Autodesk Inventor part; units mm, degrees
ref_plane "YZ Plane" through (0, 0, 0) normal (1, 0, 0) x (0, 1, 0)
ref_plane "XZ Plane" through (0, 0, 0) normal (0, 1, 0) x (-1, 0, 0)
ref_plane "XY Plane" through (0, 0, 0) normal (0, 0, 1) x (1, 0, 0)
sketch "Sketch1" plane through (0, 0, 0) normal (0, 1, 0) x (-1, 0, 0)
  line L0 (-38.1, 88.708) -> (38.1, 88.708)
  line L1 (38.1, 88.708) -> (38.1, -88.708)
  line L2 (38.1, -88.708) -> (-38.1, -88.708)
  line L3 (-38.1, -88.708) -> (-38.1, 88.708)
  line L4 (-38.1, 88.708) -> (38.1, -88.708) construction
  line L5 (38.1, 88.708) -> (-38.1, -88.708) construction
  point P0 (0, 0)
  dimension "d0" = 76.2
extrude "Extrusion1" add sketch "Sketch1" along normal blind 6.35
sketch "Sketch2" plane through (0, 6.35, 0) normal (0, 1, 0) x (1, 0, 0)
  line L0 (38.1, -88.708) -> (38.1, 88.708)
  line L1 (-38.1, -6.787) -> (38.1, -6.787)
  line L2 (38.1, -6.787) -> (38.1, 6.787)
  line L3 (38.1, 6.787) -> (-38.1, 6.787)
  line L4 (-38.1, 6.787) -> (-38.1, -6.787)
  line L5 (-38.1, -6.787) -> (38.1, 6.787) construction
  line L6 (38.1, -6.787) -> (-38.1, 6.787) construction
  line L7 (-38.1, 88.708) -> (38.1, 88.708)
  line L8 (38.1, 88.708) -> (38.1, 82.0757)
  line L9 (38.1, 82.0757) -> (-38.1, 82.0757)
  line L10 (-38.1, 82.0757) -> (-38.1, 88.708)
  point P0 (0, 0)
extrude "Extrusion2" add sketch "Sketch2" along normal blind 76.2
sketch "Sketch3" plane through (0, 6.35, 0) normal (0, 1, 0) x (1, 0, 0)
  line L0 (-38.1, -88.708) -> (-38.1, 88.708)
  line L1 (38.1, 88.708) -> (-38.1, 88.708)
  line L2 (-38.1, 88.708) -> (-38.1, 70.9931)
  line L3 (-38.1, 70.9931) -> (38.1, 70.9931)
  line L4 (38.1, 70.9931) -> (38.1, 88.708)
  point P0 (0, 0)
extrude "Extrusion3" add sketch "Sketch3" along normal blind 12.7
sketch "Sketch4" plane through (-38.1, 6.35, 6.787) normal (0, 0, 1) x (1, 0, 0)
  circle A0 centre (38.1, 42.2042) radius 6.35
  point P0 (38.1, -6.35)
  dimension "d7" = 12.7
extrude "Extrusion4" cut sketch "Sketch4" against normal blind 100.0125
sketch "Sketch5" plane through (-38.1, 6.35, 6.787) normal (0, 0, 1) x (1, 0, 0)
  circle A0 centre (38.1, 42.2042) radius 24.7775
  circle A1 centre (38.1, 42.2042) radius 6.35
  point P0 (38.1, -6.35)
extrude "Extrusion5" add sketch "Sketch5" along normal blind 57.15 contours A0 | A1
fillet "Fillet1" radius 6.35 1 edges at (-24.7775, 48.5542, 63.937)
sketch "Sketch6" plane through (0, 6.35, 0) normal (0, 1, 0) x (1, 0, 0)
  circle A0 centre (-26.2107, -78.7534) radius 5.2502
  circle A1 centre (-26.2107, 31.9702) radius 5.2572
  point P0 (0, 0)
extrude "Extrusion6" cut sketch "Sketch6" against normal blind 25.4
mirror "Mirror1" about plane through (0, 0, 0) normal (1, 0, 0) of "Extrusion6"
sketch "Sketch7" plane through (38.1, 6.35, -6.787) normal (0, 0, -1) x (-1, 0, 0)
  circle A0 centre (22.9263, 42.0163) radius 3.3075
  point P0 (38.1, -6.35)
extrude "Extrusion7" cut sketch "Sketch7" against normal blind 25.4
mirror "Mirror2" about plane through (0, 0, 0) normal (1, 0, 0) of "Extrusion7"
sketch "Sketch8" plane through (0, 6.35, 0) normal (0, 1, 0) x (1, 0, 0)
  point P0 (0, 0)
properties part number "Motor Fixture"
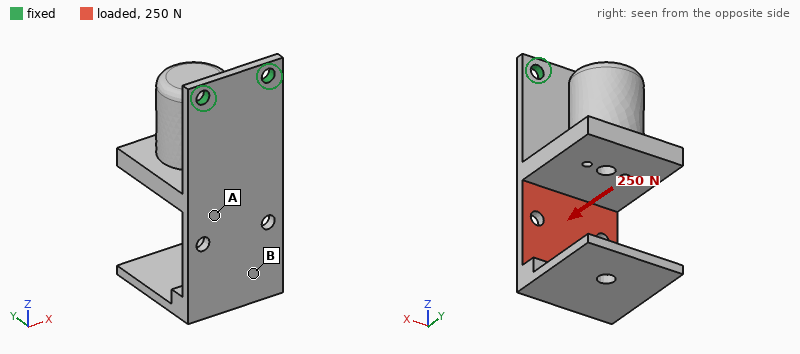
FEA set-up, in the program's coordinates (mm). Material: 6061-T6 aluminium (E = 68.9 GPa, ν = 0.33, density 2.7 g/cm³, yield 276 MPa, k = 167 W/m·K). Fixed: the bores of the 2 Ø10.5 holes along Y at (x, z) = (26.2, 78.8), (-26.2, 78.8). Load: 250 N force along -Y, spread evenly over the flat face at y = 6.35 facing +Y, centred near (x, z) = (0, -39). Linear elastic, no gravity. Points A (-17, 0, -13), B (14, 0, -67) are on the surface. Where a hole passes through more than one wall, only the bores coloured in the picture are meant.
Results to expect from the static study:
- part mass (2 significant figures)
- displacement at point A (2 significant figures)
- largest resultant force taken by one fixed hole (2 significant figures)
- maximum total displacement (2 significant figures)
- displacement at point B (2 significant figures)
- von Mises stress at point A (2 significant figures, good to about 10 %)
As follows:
850 g
0.75 mm
130 N
2.1 mm
1.5 mm
11 MPa
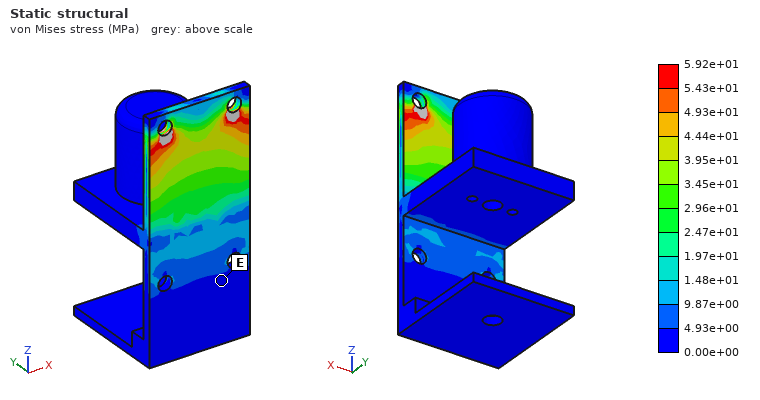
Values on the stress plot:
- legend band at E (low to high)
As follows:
0.00e+00 to 4.93e+00 MPa
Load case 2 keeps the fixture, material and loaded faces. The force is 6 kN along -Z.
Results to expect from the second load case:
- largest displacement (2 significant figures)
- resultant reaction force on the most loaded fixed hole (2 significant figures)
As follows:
2.4 mm
3.1 kN
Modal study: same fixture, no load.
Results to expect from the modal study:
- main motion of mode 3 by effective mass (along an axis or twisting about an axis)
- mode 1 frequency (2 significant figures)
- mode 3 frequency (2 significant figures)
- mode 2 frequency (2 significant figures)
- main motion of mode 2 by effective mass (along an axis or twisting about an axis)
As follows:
along Y
88 Hz
370 Hz
240 Hz
along X
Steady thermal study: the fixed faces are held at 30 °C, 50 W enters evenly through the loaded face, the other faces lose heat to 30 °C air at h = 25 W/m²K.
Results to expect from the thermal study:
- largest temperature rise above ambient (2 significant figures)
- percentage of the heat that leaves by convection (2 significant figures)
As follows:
33 K
61 %
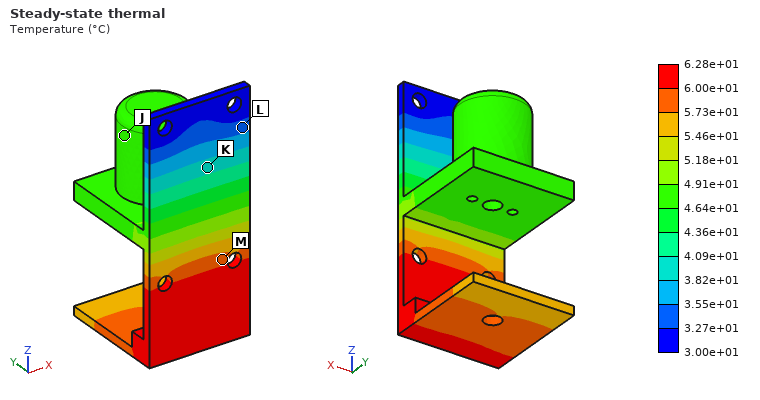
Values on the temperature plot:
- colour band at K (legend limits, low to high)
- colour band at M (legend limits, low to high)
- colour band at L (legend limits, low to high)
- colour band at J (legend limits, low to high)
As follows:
3.82e+01 to 4.09e+01 °C
5.73e+01 to 6.00e+01 °C
3.27e+01 to 3.55e+01 °C
4.64e+01 to 4.91e+01 °C
